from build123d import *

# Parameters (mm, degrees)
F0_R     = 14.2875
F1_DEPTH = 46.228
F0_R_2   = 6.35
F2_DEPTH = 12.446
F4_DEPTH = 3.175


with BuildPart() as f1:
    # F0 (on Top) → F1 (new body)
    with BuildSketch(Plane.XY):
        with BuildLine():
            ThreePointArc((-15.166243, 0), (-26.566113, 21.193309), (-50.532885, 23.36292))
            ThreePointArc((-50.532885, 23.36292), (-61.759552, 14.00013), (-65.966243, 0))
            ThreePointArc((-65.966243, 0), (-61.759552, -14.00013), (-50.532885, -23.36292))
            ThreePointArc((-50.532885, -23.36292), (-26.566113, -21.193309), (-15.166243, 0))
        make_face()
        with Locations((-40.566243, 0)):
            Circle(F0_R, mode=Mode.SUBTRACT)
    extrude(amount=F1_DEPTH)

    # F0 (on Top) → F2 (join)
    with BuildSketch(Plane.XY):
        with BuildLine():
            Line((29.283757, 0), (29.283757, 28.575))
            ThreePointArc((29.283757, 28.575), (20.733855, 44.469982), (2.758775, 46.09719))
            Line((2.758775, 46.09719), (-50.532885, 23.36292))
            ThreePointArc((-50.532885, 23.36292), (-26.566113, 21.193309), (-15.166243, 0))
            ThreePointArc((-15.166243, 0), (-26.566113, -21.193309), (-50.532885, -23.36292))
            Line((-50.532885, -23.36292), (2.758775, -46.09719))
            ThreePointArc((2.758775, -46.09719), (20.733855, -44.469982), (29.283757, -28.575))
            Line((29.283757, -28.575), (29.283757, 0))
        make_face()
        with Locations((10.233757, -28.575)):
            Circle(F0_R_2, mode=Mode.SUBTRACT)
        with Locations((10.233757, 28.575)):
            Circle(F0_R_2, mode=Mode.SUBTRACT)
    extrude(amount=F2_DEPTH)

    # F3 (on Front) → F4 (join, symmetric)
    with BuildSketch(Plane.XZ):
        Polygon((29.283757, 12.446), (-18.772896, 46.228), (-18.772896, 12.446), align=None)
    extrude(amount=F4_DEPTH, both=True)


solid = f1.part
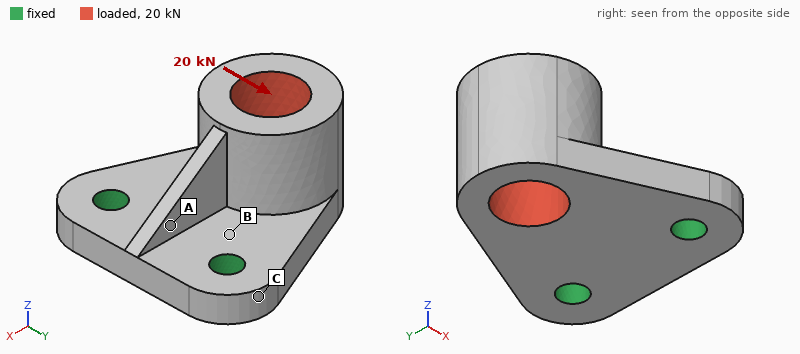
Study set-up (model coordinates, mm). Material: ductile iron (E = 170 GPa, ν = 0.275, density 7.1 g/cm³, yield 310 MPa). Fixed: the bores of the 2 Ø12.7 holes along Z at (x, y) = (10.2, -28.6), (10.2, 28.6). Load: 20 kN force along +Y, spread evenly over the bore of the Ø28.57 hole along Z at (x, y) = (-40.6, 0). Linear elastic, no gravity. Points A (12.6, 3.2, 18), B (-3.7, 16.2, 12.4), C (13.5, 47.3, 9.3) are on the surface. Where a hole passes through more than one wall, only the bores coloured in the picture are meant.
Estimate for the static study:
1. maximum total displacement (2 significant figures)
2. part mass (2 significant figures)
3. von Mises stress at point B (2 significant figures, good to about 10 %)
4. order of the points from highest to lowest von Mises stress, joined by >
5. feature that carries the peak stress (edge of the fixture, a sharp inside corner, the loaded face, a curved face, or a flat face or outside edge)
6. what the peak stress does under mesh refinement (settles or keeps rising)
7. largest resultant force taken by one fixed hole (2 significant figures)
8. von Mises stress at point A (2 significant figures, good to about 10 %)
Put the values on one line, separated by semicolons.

0.10 mm; 870 g; 87 MPa; B > A > C; edge of the fixture; keeps rising; 19 kN; 50 MPa
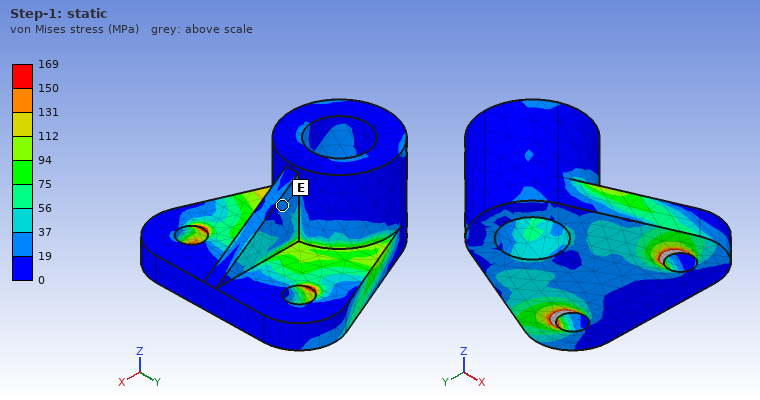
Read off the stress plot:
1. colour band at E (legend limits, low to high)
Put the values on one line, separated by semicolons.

19 to 37 MPa
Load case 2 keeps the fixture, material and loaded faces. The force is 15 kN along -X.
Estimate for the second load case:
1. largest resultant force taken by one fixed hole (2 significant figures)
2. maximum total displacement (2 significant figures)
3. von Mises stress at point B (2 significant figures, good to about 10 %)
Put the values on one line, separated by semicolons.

7.6 kN; 0.15 mm; 69 MPa
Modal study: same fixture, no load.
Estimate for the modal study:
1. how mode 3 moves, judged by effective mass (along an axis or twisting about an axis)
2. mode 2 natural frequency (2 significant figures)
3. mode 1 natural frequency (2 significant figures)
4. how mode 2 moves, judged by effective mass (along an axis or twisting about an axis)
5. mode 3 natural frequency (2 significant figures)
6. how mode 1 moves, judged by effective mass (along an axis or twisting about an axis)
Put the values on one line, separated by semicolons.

along Y; 3600 Hz; 1700 Hz; along Y; 6800 Hz; along Z
